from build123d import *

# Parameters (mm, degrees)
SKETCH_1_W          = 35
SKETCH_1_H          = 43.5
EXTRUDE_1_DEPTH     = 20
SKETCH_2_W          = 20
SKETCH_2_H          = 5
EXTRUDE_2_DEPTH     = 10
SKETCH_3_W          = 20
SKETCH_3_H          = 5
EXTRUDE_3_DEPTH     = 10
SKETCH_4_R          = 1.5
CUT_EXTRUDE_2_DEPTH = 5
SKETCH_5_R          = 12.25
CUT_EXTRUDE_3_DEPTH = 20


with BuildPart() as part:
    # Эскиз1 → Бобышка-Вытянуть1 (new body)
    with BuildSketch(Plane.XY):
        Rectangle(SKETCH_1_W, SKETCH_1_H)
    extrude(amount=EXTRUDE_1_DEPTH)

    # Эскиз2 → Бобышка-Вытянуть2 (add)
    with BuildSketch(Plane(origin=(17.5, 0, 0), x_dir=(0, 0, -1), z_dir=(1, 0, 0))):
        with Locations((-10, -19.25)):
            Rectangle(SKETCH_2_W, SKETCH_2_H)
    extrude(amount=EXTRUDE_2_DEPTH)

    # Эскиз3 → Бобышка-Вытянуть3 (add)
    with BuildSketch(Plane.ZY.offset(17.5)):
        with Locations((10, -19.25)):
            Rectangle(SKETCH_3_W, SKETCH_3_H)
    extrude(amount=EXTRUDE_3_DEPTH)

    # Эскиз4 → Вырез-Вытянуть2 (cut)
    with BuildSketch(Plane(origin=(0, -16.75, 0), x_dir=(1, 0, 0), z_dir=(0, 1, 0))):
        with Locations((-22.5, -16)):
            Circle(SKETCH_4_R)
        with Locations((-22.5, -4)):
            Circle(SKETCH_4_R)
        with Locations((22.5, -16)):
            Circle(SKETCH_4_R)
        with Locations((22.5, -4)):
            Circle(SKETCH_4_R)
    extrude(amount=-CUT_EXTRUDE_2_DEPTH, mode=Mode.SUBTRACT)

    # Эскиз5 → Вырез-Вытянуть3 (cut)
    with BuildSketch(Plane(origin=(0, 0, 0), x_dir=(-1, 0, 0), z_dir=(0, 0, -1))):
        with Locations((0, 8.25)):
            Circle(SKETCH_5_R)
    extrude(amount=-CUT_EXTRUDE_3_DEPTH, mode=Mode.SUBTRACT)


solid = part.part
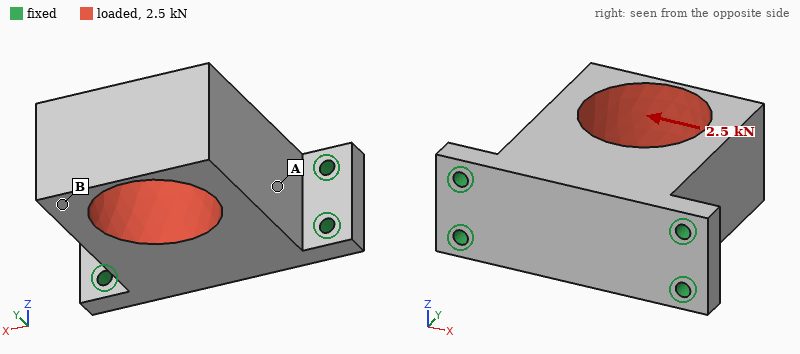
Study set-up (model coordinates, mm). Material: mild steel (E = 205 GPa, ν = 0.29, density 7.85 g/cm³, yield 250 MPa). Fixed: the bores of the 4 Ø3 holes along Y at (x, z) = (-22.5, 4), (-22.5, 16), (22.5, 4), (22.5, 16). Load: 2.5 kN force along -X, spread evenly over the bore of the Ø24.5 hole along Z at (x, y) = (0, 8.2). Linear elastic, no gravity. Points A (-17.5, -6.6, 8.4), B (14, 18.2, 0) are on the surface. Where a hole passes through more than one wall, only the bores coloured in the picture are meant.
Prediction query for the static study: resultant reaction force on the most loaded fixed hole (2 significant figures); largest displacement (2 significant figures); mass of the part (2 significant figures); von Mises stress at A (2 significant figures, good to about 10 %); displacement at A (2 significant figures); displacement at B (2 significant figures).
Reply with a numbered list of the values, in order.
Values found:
1. 1.1 kN
2. 26 µm
3. 180 g
4. 28 MPa
5. 4.8 µm
6. 22 µm
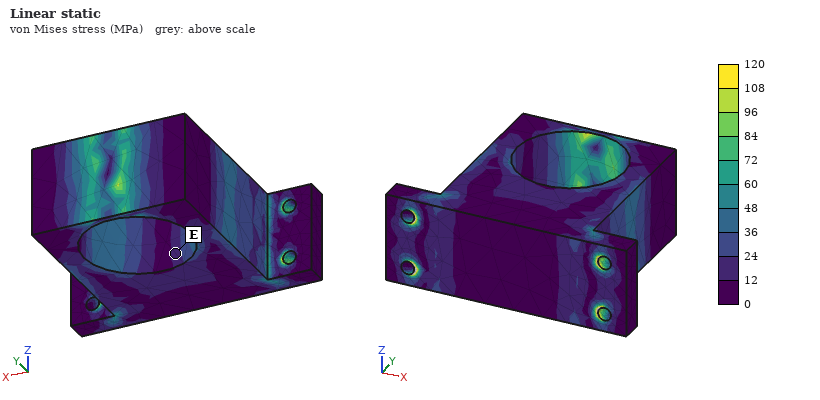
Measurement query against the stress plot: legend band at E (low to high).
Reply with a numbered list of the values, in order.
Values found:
1. 12 to 24 MPa
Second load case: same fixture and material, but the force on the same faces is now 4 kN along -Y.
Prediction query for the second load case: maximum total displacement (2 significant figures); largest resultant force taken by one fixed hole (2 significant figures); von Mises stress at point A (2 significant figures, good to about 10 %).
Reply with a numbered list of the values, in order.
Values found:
1. 11 µm
2. 1.1 kN
3. 18 MPa
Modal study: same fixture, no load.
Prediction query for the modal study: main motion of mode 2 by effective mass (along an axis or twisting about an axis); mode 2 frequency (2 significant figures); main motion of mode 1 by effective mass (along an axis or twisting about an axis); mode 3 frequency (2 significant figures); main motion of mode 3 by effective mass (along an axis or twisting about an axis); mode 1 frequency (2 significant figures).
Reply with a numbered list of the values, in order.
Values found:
1. along X
2. 6600 Hz
3. along Z
4. 11 kHz
5. twisting about Y
6. 3800 Hz
